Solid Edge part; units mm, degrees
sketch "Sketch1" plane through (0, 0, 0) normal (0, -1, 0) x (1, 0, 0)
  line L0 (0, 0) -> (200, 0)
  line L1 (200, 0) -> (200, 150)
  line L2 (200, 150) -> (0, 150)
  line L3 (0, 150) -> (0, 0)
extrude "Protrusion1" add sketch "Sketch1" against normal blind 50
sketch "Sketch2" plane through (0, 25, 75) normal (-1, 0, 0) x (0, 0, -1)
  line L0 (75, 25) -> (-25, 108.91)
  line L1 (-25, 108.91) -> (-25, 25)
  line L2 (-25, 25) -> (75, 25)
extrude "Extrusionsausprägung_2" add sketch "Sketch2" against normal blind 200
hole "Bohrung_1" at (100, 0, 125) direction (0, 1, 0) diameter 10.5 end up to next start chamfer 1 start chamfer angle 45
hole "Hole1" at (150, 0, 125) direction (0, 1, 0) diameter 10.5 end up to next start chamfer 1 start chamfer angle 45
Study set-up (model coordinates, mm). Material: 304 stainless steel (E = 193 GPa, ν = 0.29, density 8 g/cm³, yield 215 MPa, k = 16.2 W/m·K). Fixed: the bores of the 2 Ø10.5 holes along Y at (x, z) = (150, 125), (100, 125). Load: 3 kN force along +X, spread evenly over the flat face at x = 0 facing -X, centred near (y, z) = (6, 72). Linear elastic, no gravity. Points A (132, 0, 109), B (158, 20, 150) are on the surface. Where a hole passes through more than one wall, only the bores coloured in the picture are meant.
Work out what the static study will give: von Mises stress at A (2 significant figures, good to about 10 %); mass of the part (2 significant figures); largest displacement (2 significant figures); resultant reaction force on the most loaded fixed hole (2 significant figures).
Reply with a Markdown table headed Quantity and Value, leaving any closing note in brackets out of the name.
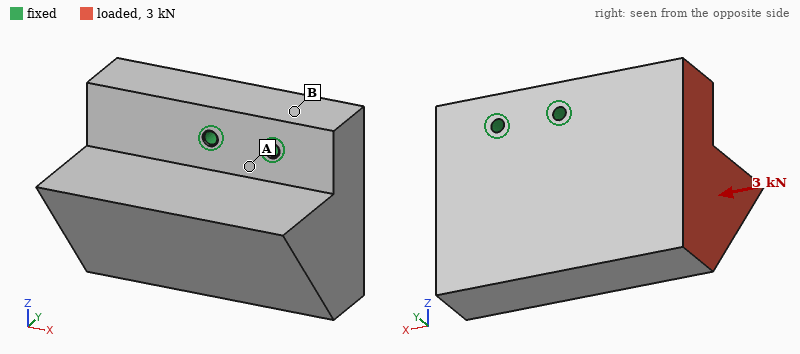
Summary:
| Quantity | Value |
|---|---|
| von Mises stress at A | 2.1 MPa |
| mass of the part | 19 kg |
| largest displacement | 2.3 µm |
| resultant reaction force on the most loaded fixed hole | 3.3 kN |
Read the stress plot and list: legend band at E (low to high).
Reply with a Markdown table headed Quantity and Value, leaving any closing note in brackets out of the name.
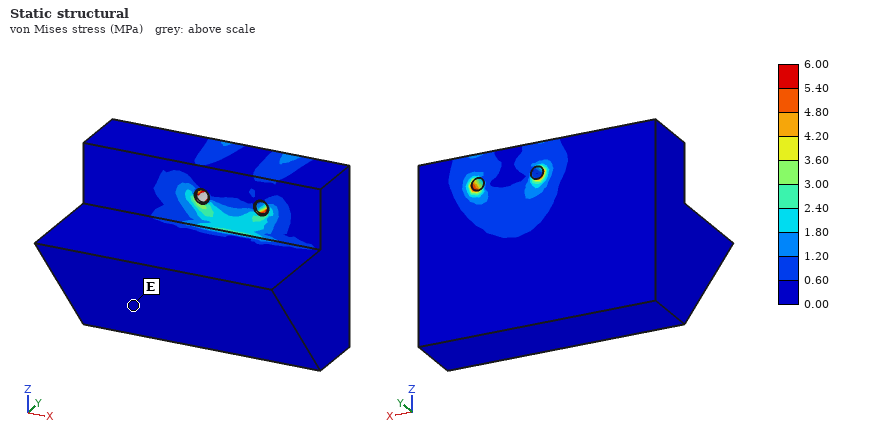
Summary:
| Quantity | Value |
|---|---|
| legend band at E | 0.00 to 0.60 MPa |
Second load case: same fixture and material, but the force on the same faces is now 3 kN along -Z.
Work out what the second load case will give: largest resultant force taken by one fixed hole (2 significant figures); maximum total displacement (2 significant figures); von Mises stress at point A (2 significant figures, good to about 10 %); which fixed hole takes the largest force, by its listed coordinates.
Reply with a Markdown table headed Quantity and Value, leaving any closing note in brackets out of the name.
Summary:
| Quantity | Value |
|---|---|
| largest resultant force taken by one fixed hole | 8.0 kN |
| maximum total displacement | 5.8 µm |
| von Mises stress at point A | 1.8 MPa |
| which fixed hole takes the largest force, by its listed coordinates | (100, 125) |
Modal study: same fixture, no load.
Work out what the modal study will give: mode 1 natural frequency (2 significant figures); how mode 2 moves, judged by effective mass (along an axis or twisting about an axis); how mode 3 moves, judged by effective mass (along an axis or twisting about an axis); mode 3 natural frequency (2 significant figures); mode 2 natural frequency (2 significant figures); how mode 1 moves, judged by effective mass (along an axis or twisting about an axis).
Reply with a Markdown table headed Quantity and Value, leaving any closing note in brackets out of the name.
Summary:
| Quantity | Value |
|---|---|
| mode 1 natural frequency | 1200 Hz |
| how mode 2 moves, judged by effective mass | along X |
| how mode 3 moves, judged by effective mass | twisting about Z |
| mode 3 natural frequency | 1900 Hz |
| mode 2 natural frequency | 1500 Hz |
| how mode 1 moves, judged by effective mass | along Y |
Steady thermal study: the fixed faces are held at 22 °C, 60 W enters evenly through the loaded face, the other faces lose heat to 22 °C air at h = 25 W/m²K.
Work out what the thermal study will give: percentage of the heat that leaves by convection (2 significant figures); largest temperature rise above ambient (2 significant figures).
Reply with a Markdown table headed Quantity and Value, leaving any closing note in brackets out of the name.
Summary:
| Quantity | Value |
|---|---|
| percentage of the heat that leaves by convection | 58 % |
| largest temperature rise above ambient | 35 K |
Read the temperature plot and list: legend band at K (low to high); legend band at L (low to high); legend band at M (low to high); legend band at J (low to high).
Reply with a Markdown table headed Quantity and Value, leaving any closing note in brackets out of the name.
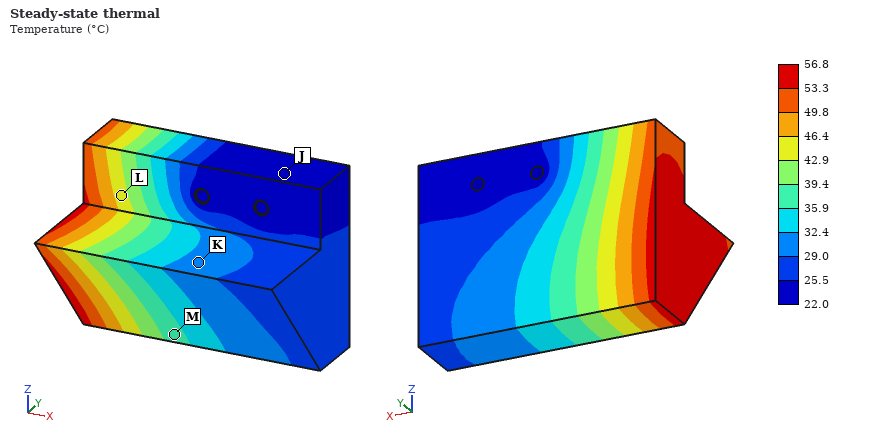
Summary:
| Quantity | Value |
|---|---|
| legend band at K | 29.0 to 32.4 °C |
| legend band at L | 42.9 to 46.4 °C |
| legend band at M | 35.9 to 39.4 °C |
| legend band at J | 22.0 to 25.5 °C |
